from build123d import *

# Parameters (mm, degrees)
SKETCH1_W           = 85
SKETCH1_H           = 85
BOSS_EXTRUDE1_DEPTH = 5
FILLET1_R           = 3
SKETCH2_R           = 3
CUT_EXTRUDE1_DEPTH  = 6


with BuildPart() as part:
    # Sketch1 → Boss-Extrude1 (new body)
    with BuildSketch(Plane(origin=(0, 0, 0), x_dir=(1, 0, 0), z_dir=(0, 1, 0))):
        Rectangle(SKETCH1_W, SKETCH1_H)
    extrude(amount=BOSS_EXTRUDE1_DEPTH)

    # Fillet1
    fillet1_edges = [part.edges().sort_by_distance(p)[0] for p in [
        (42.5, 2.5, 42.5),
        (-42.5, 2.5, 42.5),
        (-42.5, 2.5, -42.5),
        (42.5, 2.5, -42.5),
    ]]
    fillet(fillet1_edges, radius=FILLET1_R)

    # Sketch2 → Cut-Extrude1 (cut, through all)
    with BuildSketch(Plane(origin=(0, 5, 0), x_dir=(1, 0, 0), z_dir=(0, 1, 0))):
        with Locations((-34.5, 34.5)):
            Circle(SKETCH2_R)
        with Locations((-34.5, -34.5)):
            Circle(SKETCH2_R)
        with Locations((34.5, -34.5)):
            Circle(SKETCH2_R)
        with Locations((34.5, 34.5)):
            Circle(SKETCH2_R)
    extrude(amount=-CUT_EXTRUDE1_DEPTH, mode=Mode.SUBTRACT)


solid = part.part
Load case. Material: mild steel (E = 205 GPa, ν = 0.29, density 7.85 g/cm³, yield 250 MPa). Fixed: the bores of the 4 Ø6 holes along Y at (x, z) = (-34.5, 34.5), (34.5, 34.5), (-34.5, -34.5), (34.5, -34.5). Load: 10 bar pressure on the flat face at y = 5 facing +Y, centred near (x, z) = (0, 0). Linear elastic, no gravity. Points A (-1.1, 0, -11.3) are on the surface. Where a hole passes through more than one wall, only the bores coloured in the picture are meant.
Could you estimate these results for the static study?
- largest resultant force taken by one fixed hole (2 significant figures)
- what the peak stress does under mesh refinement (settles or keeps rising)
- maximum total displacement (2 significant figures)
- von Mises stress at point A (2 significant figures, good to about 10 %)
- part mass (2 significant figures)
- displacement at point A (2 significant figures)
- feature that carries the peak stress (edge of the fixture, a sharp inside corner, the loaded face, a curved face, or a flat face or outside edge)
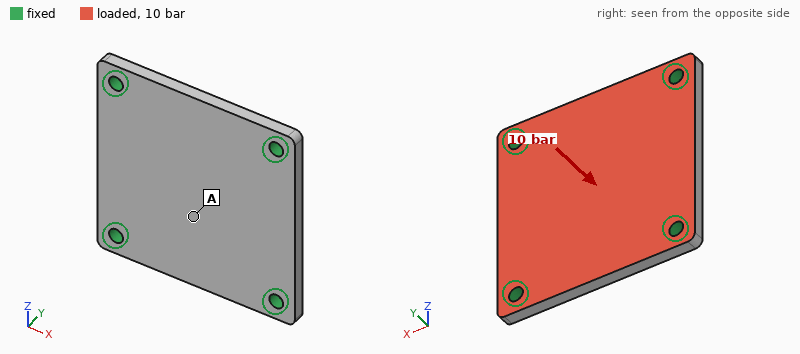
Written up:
1.8 kN
keeps rising
68 µm
54 MPa
280 g
63 µm
edge of the fixture
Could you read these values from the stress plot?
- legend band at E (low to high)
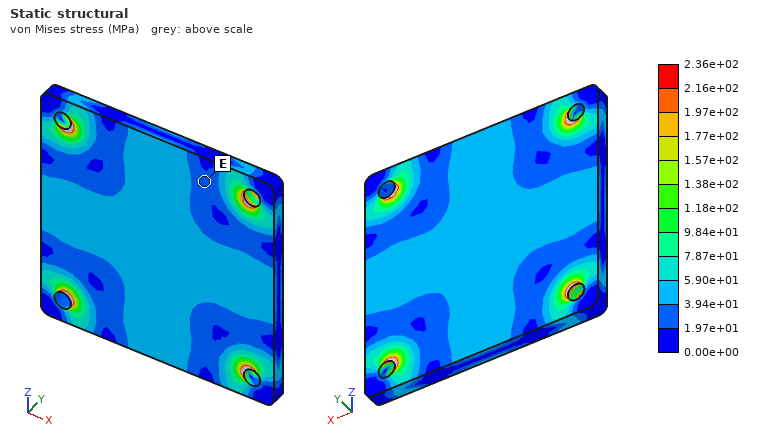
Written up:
1.97e+01 to 3.94e+01 MPa
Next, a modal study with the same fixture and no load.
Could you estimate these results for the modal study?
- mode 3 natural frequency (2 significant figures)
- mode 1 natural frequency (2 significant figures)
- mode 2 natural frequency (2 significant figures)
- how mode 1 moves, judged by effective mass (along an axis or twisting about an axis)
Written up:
6200 Hz
3800 Hz
6200 Hz
along Y
